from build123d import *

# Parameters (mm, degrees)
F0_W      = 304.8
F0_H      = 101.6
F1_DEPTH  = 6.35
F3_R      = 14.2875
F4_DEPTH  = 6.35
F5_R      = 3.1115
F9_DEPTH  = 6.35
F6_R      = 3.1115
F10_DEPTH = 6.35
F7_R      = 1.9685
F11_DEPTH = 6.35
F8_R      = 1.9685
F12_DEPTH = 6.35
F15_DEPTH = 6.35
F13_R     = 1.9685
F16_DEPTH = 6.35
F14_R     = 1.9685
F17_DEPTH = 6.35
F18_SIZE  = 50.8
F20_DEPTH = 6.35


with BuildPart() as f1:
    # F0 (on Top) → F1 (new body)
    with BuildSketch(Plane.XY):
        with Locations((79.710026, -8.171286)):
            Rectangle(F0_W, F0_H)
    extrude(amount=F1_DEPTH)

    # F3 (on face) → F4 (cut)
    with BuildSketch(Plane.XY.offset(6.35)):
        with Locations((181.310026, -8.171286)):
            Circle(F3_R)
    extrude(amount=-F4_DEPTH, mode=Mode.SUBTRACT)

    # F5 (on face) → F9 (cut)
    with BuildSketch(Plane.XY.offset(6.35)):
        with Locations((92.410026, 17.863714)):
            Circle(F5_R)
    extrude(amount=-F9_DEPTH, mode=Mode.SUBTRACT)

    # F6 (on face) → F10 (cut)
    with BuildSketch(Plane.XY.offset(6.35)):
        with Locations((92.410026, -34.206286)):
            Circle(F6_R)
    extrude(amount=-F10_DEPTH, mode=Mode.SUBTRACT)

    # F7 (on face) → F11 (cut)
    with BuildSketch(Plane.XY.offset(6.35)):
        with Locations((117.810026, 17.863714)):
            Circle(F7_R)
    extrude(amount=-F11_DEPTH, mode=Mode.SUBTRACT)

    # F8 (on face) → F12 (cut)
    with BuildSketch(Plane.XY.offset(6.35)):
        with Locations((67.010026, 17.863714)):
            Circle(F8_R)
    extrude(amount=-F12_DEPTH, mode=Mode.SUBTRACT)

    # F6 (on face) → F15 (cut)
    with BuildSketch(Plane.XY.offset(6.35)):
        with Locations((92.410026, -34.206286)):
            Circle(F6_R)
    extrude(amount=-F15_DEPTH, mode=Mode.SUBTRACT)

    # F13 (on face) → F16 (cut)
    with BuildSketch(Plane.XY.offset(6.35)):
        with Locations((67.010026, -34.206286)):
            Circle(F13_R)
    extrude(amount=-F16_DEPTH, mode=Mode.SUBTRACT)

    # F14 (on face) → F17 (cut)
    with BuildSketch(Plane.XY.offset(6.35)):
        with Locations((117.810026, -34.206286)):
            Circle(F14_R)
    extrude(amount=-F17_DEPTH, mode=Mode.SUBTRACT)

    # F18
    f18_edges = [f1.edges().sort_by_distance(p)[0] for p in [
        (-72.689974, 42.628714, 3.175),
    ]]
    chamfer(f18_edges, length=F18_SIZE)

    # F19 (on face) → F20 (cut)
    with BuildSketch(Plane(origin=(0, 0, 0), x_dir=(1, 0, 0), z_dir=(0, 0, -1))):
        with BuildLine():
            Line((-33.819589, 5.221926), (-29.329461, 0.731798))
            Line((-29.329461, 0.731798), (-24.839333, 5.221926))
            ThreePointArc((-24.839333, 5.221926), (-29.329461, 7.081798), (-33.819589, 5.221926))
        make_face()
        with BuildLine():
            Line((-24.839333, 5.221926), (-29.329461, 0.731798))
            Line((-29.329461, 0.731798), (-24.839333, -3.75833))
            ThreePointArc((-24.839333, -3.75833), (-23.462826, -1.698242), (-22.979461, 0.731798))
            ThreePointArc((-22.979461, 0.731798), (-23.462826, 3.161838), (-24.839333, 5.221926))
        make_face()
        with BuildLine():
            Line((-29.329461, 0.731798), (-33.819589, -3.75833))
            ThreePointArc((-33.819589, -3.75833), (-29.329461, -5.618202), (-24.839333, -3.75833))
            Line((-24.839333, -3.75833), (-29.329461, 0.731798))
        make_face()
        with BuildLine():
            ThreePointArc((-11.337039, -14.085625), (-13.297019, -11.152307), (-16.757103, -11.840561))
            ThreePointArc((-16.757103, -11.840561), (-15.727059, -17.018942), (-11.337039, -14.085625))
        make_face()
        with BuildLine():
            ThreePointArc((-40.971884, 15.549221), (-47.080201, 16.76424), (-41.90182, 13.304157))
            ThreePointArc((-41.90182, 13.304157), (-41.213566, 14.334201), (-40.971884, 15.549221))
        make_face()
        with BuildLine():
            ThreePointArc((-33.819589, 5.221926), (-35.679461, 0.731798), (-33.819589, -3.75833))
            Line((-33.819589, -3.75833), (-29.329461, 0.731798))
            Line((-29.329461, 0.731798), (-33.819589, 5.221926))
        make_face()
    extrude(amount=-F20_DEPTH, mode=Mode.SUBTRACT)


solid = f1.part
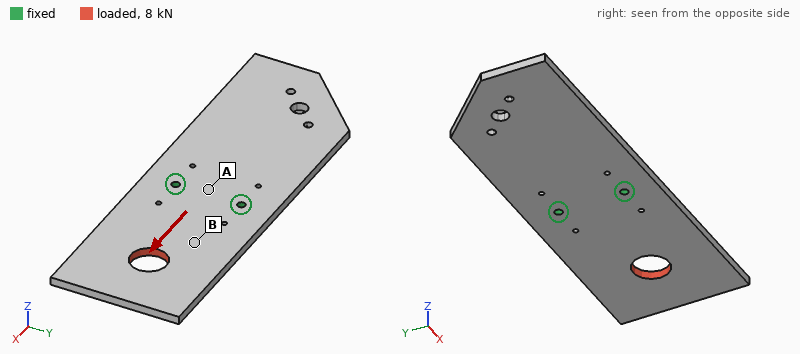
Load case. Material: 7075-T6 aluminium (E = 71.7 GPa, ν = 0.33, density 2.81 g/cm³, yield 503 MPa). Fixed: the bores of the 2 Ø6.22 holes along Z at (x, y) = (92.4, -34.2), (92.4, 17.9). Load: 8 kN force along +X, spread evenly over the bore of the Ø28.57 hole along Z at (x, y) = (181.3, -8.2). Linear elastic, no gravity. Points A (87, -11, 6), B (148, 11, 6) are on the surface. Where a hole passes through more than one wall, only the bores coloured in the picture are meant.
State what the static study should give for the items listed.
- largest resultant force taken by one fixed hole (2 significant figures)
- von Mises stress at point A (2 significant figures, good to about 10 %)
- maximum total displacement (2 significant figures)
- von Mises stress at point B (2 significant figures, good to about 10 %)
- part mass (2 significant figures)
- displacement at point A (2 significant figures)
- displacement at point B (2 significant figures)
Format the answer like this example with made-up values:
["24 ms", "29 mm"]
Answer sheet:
["4.0 kN", "5.1 MPa", "28 µm", "15 MPa", "510 g", "4.2 µm", "13 µm"]
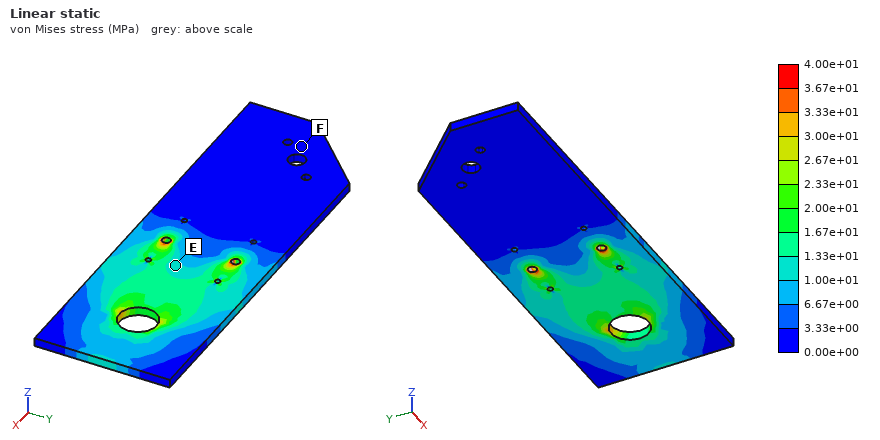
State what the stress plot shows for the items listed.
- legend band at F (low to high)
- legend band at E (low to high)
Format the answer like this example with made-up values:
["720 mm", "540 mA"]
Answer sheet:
["0.00e+00 to 3.33e+00 MPa", "1.00e+01 to 1.33e+01 MPa"]
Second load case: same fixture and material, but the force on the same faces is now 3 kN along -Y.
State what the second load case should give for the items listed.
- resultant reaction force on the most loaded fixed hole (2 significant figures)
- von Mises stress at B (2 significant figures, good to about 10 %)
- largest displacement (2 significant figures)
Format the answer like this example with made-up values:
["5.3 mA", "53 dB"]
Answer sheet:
["5.1 kN", "10 MPa", "88 µm"]
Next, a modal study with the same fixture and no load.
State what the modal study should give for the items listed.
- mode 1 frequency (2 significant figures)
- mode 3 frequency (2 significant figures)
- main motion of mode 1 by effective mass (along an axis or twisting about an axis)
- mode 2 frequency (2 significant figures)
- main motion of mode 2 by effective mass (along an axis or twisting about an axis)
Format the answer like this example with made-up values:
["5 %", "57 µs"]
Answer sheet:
["210 Hz", "760 Hz", "along Z", "270 Hz", "along Z"]
